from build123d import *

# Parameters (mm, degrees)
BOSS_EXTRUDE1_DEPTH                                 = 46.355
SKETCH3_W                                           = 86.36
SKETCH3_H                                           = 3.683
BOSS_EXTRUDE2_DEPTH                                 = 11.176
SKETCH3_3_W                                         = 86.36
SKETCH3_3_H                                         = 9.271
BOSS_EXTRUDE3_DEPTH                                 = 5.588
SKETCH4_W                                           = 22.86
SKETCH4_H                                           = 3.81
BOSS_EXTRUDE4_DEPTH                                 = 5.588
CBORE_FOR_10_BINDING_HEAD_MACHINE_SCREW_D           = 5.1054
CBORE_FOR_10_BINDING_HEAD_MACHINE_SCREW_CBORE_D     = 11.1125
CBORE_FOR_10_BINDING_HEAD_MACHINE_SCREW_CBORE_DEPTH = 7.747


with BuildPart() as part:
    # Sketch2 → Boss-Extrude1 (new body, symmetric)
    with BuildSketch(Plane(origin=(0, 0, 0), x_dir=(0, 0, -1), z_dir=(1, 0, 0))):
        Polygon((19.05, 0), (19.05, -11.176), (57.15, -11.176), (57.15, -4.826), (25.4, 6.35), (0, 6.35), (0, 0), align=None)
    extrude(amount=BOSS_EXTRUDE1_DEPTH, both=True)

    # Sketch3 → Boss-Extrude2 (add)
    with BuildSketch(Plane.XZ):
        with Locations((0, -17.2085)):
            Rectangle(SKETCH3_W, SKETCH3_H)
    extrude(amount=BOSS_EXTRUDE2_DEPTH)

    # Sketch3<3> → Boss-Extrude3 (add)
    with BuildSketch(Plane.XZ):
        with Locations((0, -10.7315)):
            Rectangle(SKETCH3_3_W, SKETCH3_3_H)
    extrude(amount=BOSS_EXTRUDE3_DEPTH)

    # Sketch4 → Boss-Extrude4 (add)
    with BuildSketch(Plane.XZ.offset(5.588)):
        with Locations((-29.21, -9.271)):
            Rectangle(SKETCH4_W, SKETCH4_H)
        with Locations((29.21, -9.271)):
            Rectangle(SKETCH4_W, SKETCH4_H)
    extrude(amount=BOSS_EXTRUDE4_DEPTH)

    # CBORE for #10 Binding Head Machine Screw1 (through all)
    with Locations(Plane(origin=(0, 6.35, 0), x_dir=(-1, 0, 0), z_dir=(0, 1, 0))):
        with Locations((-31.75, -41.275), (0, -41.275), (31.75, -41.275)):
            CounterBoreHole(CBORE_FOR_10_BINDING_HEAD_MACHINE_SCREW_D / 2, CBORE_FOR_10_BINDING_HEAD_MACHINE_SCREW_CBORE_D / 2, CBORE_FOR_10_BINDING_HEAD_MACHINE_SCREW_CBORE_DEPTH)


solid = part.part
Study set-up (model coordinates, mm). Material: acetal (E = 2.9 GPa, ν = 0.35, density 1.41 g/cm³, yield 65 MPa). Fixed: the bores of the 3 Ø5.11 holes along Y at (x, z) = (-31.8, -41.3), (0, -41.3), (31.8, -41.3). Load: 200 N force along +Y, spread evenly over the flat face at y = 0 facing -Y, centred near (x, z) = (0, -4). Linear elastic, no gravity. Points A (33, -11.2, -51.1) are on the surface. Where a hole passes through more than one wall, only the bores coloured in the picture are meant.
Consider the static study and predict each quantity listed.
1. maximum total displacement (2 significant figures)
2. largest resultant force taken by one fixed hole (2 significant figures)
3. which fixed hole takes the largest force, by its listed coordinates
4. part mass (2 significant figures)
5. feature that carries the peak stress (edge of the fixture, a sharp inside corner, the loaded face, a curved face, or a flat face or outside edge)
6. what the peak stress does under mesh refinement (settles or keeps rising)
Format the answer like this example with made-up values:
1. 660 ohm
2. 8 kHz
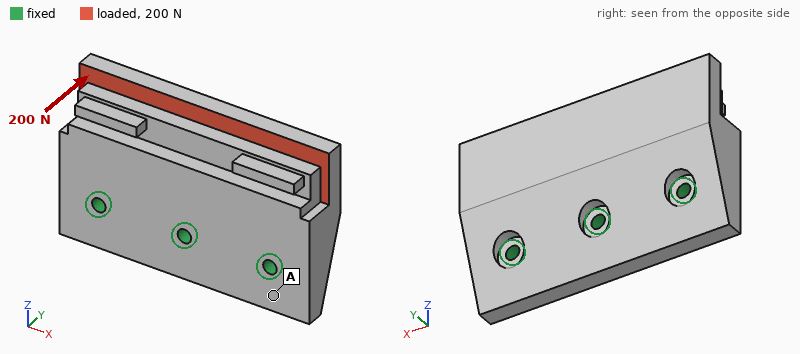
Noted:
1. 0.15 mm
2. 73 N
3. (0, -41.3)
4. 91 g
5. edge of the fixture
6. keeps rising
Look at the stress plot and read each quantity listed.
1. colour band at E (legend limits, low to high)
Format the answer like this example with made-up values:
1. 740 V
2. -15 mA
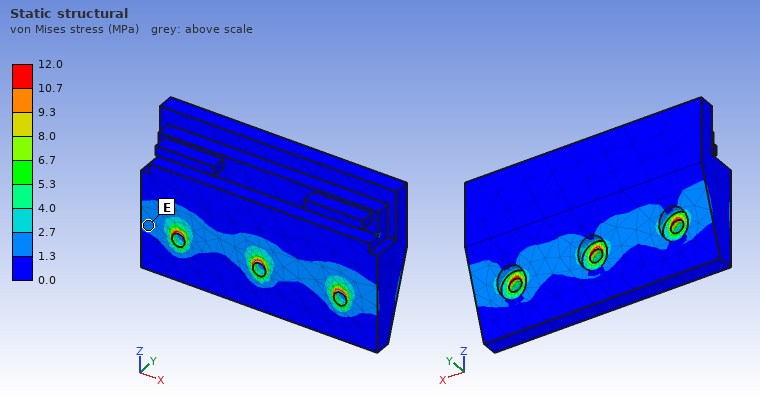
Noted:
1. 1.3 to 2.7 MPa
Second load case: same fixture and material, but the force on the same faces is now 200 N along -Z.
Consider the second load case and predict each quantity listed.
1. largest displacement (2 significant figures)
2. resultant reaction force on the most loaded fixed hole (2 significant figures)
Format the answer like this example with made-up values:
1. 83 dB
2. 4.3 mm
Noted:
1. 20 µm
2. 72 N
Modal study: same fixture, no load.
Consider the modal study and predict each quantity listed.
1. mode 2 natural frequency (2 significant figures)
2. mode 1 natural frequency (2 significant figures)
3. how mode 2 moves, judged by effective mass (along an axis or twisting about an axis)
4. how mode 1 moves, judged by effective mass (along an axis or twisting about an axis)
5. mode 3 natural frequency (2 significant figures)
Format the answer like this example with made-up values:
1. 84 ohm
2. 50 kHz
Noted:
1. 2000 Hz
2. 1300 Hz
3. twisting about Z
4. along Y
5. 3600 Hz
